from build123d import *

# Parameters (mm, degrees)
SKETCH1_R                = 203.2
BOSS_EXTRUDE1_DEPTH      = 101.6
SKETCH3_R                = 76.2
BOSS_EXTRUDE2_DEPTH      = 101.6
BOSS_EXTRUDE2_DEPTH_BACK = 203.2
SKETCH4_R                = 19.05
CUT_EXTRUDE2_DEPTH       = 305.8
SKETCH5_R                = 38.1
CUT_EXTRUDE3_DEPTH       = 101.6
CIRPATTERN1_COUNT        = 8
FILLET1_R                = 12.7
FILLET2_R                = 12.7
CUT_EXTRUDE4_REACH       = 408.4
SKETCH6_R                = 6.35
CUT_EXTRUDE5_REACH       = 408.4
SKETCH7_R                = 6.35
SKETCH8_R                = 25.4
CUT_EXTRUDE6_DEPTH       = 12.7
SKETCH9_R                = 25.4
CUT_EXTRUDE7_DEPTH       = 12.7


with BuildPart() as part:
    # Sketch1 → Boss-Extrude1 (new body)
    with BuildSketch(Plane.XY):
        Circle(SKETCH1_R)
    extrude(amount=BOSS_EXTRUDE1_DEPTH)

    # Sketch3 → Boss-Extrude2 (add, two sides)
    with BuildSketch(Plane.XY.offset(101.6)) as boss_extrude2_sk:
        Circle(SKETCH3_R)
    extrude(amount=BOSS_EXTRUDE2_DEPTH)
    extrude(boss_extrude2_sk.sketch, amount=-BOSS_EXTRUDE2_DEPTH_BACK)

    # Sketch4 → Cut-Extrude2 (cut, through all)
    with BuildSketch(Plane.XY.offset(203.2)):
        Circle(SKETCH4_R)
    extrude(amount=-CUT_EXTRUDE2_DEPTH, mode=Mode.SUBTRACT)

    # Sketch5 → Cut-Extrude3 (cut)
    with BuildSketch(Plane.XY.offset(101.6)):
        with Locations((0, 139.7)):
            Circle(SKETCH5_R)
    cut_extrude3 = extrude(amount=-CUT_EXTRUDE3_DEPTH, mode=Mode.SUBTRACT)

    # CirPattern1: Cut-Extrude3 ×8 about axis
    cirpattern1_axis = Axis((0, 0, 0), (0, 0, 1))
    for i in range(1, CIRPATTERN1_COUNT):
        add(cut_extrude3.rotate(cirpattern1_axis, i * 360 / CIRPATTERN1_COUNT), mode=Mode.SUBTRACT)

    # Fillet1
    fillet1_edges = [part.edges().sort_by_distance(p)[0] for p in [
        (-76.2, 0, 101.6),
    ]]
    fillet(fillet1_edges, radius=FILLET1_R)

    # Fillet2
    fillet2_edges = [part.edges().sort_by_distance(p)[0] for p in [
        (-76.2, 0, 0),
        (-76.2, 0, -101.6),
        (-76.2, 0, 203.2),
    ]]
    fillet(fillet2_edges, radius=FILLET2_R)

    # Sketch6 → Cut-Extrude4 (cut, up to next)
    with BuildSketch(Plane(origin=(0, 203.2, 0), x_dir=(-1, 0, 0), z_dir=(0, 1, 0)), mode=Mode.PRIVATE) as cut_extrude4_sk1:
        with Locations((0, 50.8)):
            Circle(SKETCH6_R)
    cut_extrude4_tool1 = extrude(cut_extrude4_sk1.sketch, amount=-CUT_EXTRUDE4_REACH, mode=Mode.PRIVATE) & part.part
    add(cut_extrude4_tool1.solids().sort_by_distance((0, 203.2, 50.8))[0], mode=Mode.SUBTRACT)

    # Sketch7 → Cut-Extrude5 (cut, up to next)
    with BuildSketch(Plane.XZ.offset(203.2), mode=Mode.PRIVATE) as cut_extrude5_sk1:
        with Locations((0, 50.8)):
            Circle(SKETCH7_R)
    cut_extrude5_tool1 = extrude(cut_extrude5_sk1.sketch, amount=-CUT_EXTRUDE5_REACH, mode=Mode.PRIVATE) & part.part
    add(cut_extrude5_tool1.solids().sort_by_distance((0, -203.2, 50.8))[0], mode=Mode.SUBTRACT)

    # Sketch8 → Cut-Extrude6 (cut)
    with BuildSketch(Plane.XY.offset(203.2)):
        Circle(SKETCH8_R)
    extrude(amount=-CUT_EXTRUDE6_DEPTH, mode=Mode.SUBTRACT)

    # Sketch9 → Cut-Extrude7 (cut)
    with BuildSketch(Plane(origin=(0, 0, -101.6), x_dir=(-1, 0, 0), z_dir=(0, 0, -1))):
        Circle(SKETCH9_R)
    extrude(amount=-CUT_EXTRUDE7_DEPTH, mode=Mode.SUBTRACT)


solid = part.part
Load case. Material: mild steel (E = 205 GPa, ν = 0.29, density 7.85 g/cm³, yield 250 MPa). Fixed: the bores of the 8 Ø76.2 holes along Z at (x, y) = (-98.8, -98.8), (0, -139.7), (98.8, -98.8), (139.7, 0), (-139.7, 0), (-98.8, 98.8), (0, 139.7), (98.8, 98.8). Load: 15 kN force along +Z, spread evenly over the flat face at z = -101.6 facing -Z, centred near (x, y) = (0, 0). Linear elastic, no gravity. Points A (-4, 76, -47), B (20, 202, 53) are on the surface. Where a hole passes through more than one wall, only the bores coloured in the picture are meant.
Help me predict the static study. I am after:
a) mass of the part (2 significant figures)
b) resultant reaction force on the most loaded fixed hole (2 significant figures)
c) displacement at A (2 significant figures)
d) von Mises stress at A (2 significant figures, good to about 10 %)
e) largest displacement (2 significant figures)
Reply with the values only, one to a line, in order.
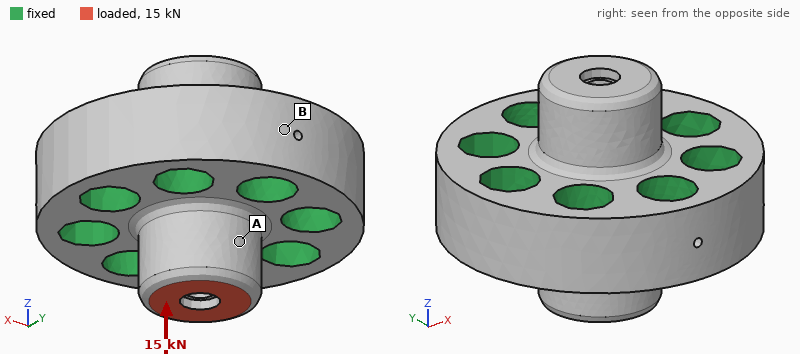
100 kg
2.1 kN
0.43 µm
0.73 MPa
0.74 µm
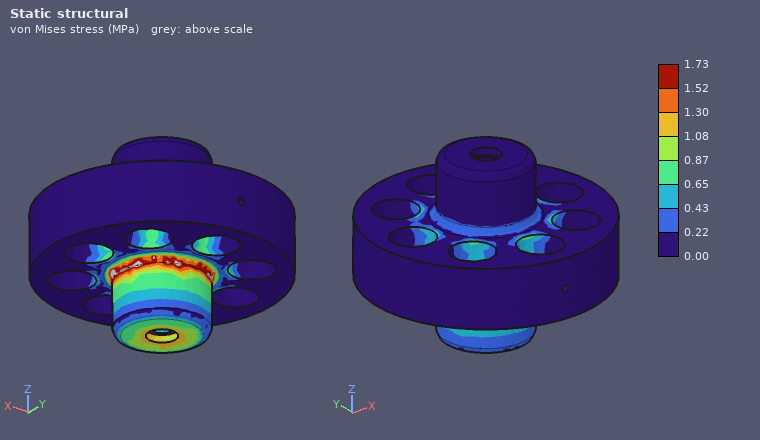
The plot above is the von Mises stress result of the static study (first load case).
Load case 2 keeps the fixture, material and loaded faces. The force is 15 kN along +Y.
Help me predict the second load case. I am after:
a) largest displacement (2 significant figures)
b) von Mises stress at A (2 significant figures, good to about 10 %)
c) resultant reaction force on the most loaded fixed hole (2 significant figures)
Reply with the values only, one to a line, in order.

3.8 µm
2.5 MPa
6.1 kN
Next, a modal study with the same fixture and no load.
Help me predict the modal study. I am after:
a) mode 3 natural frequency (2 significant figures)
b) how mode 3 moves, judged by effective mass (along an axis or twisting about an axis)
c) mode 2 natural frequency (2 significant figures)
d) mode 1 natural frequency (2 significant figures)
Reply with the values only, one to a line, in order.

4900 Hz
along Y
4500 Hz
4500 Hz
